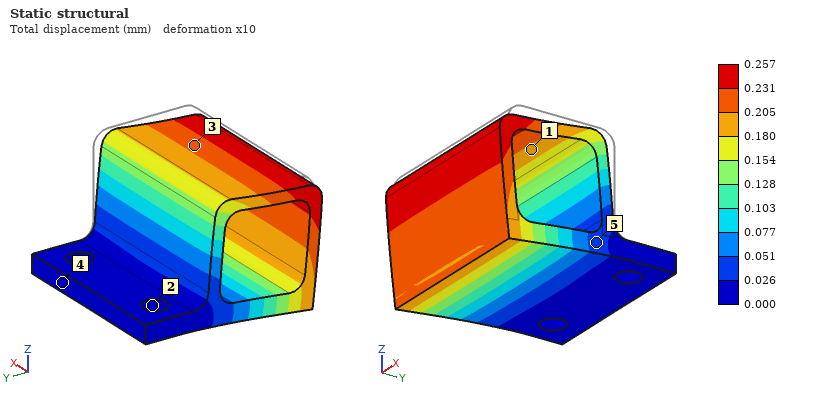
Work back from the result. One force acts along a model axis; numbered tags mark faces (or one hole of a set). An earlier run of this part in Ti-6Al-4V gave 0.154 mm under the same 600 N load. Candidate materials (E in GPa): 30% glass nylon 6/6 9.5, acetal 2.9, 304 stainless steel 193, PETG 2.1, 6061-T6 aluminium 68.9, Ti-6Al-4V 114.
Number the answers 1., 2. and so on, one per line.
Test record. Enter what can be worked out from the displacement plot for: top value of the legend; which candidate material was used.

1. 0.257 mm
2. 6061-T6 aluminium
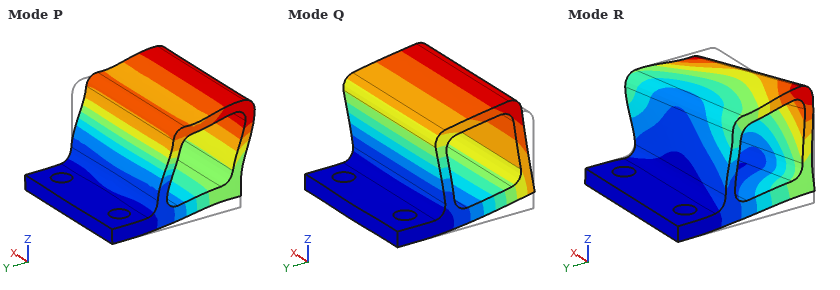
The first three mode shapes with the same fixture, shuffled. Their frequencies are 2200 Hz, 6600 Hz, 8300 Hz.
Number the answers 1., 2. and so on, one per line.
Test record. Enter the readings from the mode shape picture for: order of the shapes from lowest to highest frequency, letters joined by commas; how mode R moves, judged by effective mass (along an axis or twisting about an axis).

1. Q, R, P
2. along X
